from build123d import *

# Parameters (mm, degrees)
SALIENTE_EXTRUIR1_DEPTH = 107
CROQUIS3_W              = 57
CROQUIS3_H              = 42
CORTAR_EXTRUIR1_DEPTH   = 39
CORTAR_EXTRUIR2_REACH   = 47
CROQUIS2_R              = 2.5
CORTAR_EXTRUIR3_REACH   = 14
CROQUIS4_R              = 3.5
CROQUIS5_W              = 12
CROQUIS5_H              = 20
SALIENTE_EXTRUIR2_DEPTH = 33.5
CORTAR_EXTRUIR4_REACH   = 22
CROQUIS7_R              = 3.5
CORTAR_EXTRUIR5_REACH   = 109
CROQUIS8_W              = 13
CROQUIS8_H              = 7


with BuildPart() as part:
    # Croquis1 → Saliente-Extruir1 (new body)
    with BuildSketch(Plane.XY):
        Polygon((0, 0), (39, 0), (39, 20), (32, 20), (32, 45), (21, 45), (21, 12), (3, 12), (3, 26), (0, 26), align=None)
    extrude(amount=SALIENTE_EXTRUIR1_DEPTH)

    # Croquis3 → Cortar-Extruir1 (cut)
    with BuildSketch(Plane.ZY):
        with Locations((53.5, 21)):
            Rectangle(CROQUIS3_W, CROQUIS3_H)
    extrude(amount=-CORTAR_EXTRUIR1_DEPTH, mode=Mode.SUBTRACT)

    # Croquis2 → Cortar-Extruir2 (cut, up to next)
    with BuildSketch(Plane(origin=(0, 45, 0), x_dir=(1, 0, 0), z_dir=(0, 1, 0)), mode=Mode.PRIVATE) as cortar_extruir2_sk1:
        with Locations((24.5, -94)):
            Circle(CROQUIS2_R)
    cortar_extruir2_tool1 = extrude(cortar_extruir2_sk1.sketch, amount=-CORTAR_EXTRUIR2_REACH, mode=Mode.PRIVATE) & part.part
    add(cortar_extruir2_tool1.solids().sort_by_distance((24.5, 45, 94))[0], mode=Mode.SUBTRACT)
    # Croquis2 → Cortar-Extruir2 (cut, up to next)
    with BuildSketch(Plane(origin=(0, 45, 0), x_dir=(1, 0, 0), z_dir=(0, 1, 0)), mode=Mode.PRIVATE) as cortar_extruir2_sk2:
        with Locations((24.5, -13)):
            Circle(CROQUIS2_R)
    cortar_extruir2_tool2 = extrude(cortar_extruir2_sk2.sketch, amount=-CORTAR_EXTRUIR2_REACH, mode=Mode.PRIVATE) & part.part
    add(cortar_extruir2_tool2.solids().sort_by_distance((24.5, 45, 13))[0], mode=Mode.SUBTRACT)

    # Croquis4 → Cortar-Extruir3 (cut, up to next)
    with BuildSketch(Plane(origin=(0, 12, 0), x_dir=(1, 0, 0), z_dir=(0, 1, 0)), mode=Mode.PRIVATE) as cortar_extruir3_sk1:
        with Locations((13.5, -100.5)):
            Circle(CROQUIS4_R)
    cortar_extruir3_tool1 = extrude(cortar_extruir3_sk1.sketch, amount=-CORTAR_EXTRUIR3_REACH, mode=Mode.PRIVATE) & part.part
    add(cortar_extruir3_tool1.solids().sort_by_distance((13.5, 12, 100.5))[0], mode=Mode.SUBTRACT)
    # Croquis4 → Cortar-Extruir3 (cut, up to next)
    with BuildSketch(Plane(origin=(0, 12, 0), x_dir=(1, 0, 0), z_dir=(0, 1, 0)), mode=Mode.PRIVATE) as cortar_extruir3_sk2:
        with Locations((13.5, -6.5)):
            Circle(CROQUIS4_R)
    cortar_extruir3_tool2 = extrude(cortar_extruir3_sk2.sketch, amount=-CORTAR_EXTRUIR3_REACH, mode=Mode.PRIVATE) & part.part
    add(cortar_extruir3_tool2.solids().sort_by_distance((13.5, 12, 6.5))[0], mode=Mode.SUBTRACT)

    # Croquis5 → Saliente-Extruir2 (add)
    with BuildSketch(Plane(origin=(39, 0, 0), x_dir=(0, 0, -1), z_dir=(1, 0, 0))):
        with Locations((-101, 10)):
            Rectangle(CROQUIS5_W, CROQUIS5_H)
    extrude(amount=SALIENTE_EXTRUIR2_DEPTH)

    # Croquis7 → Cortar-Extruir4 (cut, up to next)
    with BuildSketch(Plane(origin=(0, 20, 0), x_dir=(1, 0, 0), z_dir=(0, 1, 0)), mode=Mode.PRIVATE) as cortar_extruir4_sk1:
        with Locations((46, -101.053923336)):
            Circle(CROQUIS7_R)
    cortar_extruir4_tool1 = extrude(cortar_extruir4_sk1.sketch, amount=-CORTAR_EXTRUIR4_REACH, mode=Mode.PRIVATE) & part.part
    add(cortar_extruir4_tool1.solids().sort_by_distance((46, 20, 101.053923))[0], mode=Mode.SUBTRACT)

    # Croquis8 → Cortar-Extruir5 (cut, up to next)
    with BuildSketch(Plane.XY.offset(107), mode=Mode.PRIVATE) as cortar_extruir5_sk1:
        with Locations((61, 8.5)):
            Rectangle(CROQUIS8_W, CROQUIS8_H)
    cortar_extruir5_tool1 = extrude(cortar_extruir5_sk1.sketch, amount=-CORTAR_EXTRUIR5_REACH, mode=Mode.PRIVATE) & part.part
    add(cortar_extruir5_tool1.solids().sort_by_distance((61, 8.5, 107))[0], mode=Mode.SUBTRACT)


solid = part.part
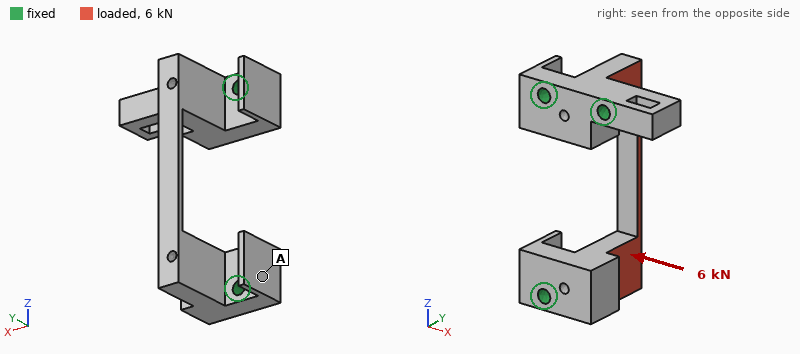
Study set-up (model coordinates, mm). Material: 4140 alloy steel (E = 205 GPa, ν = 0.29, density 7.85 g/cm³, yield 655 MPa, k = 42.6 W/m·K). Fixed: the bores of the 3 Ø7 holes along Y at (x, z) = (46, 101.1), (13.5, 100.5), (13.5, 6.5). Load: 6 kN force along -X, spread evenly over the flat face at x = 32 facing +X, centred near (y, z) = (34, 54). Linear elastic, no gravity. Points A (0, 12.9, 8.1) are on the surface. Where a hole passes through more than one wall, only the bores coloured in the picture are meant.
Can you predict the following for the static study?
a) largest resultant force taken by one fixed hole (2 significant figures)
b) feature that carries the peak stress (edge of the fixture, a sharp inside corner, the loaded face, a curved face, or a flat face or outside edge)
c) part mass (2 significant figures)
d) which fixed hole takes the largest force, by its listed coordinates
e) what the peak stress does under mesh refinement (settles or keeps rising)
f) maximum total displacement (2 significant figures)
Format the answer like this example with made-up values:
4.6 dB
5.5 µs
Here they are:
3.8 kN
edge of the fixture
410 g
(46, 101.1)
keeps rising
100 µm
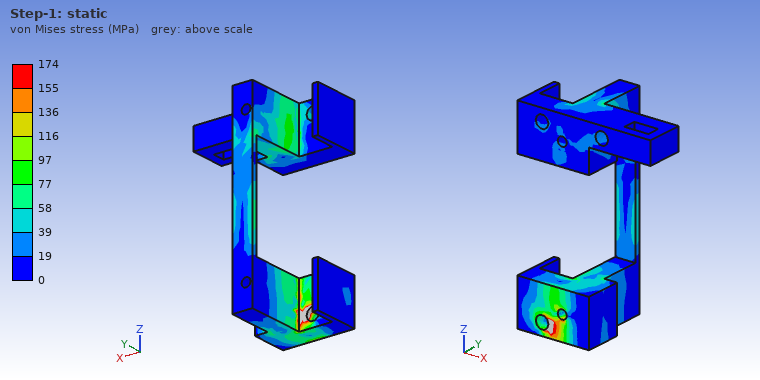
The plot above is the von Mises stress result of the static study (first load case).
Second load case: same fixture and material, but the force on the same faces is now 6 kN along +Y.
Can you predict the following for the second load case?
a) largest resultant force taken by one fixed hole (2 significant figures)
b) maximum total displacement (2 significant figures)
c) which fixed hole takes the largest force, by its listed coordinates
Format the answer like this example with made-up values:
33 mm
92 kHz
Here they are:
3.0 kN
0.12 mm
(13.5, 6.5)
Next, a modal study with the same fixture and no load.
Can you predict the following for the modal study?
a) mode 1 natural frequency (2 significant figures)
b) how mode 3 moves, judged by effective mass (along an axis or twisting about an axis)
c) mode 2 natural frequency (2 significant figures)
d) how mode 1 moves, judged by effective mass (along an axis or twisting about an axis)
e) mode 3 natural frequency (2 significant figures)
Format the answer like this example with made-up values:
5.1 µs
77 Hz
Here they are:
4100 Hz
along Z
4400 Hz
along X
5500 Hz
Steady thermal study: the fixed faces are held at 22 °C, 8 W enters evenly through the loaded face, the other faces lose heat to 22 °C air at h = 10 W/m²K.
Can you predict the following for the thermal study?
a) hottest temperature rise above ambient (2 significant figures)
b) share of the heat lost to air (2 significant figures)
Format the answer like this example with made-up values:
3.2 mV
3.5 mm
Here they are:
15 K
8.5 %
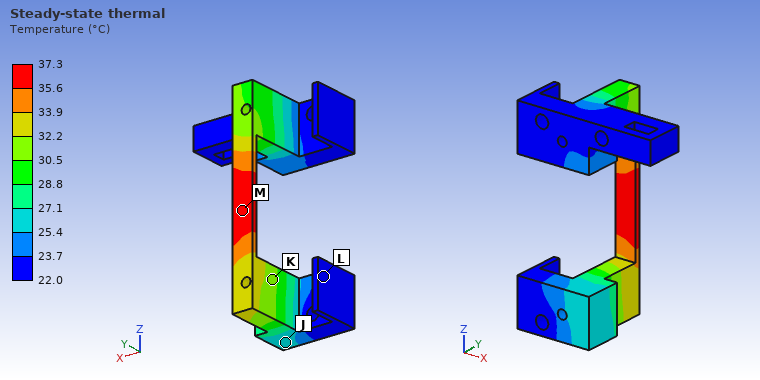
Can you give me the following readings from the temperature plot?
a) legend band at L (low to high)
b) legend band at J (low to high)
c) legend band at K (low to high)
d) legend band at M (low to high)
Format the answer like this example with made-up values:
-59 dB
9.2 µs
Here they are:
22.0 to 23.7 °C
25.4 to 27.1 °C
30.5 to 32.2 °C
35.6 to 37.3 °C
